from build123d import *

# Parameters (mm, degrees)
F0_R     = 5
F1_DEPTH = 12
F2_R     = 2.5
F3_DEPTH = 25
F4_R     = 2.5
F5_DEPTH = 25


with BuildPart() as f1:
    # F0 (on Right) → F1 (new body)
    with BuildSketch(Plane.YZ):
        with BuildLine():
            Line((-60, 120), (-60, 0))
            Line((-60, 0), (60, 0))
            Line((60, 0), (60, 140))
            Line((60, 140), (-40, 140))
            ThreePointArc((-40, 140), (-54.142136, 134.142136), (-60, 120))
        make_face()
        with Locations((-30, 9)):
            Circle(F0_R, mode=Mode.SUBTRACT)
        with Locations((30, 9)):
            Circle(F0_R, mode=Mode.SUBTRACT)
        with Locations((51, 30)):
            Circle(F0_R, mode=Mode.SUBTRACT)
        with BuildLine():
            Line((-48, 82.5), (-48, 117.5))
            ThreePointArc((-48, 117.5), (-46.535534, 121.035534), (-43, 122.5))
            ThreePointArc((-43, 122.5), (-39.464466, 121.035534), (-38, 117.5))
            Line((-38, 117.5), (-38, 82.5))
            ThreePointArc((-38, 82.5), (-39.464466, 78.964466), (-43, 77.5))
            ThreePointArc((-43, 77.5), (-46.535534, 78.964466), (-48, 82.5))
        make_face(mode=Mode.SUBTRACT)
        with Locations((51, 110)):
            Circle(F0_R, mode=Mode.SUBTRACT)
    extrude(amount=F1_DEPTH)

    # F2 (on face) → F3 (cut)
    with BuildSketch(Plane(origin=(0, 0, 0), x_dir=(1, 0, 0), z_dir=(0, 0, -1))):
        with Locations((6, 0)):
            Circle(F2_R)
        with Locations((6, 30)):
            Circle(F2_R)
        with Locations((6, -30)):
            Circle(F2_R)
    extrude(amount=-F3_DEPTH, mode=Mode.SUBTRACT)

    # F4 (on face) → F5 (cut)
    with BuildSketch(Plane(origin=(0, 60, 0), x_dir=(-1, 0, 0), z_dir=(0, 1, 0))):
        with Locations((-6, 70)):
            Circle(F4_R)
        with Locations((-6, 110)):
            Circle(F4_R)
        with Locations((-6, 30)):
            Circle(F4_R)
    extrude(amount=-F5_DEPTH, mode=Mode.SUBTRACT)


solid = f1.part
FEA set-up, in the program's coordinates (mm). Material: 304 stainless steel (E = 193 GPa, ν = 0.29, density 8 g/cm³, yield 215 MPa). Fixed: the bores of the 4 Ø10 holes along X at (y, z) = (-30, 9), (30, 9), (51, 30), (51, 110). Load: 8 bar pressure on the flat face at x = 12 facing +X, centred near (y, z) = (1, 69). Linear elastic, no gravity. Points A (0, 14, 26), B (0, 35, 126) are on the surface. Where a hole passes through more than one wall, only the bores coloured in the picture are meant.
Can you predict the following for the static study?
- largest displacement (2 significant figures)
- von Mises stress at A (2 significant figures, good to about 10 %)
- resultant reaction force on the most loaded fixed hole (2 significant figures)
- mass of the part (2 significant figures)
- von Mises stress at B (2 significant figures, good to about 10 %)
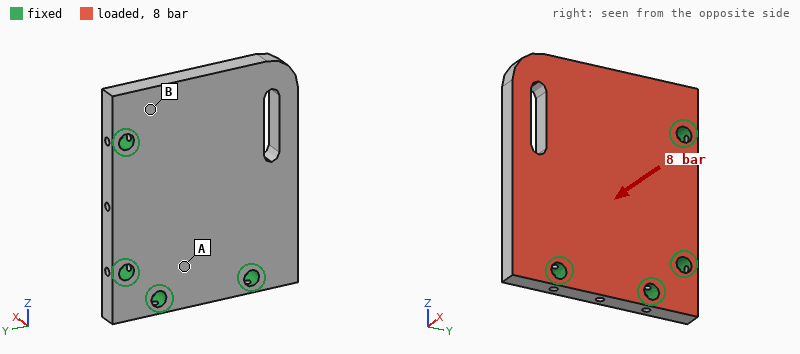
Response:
0.25 mm
29 MPa
5.7 kN
1.5 kg
56 MPa
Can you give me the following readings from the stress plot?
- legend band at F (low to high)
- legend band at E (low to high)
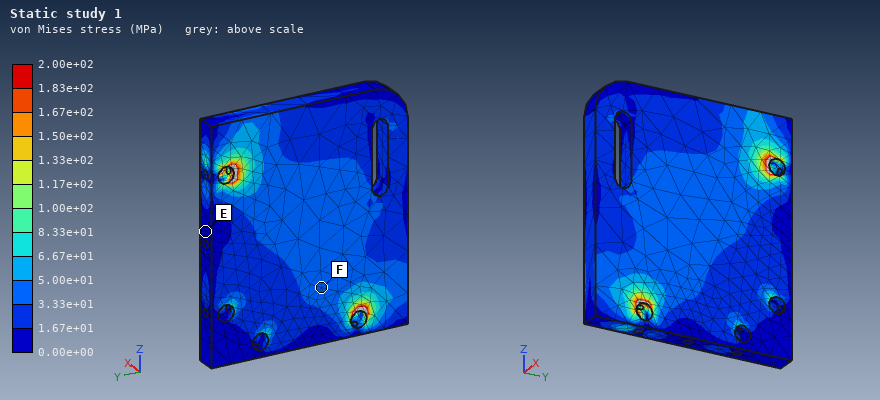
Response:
3.33e+01 to 5.00e+01 MPa
0.00e+00 to 1.67e+01 MPa
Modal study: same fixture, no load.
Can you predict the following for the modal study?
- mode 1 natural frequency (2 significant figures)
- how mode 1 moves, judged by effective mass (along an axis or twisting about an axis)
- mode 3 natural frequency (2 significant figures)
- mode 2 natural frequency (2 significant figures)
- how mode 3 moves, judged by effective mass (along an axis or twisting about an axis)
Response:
1300 Hz
along X
4600 Hz
3600 Hz
along X
